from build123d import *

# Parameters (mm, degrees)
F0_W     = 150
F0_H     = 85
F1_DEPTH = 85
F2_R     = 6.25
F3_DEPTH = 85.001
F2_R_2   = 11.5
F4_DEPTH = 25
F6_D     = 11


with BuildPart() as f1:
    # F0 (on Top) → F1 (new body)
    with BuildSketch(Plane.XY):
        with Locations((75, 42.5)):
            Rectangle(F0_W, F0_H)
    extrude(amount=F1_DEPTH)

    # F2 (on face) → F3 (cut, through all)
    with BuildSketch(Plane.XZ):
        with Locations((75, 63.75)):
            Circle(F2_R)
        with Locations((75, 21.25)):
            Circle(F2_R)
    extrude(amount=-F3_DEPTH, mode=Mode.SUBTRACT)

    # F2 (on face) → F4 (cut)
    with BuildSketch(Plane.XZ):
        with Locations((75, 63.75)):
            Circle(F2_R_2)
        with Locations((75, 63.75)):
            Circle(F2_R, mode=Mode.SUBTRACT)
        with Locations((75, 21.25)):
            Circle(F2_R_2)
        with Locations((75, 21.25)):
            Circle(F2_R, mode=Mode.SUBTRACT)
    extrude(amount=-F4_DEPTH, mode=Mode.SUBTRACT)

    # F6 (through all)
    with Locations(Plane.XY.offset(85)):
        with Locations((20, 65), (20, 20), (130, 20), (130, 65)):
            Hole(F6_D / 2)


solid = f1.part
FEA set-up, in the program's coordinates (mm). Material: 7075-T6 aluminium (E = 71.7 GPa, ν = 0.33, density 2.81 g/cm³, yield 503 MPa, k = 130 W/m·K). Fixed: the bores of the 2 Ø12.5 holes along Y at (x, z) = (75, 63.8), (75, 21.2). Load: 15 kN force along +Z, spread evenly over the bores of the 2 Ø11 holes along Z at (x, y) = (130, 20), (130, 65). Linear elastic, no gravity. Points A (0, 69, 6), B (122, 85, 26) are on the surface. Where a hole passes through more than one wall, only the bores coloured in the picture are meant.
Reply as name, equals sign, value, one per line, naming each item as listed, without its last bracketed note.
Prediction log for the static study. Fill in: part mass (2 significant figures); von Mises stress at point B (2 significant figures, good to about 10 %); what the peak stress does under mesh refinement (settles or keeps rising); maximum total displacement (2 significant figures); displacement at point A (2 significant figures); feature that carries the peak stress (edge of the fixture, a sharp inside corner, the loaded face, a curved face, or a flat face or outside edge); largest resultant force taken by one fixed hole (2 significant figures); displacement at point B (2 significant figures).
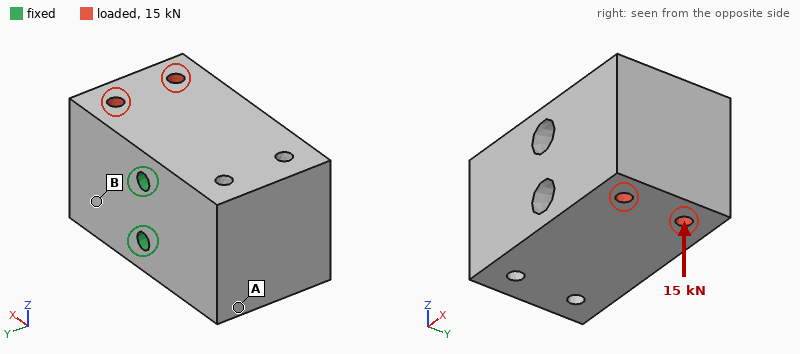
part mass = 2.9 kg
von Mises stress at point B = 4.5 MPa
what the peak stress does under mesh refinement = keeps rising
maximum total displacement = 15 µm
displacement at point A = 3.8 µm
feature that carries the peak stress = edge of the fixture
largest resultant force taken by one fixed hole = 18 kN
displacement at point B = 8.0 µm
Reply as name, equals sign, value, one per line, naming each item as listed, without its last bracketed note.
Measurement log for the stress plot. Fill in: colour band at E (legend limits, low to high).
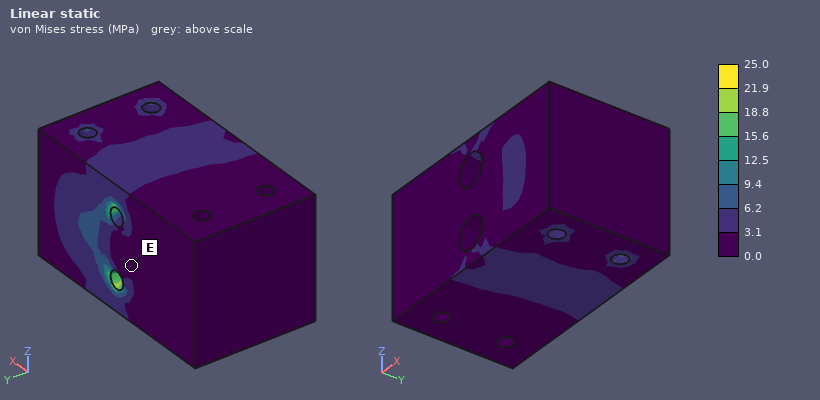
colour band at E = 0.0 to 3.1 MPa
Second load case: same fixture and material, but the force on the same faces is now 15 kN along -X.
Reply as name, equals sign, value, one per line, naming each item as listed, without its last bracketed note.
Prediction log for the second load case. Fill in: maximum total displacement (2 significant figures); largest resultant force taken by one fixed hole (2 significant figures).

maximum total displacement = 4.1 µm
largest resultant force taken by one fixed hole = 7.6 kN
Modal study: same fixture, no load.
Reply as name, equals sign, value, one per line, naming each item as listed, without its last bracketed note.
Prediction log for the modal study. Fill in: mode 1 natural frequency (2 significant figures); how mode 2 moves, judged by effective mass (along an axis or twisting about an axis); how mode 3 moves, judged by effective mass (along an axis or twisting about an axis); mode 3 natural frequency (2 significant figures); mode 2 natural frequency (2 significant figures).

mode 1 natural frequency = 4700 Hz
how mode 2 moves, judged by effective mass = twisting about Y
how mode 3 moves, judged by effective mass = along Z
mode 3 natural frequency = 6900 Hz
mode 2 natural frequency = 5400 Hz
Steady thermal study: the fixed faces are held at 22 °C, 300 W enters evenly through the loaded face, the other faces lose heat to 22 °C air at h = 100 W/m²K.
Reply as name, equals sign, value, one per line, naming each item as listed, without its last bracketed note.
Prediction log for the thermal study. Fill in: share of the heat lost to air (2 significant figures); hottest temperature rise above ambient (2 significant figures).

share of the heat lost to air = 16 %
hottest temperature rise above ambient = 20 K
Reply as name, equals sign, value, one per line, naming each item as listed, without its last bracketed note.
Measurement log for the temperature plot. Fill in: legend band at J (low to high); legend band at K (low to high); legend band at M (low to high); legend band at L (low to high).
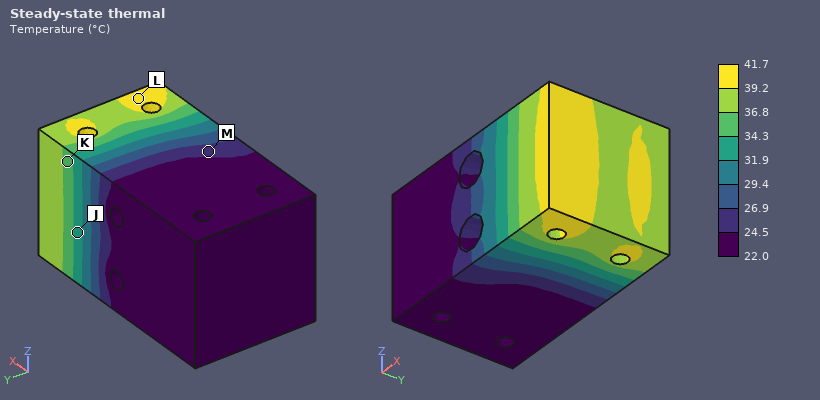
legend band at J = 31.9 to 34.3 °C
legend band at K = 34.3 to 36.8 °C
legend band at M = 24.5 to 26.9 °C
legend band at L = 39.2 to 41.7 °C
